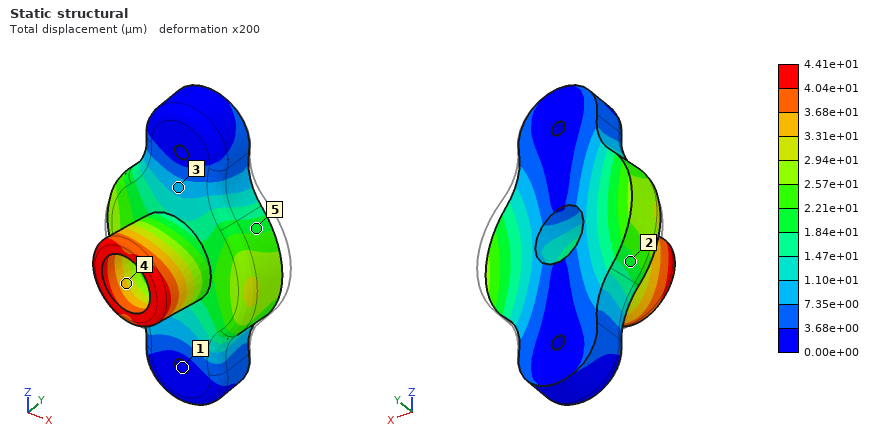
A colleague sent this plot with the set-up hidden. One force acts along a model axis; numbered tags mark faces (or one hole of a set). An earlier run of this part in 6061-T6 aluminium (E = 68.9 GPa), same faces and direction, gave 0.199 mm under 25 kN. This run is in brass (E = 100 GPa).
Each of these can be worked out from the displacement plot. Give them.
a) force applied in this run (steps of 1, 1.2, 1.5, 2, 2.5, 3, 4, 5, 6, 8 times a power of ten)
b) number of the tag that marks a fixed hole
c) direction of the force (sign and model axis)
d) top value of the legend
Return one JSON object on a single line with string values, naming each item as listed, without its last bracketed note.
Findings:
{"force applied in this run": "8 kN", "number of the tag that marks a fixed hole": "1", "direction of the force": "-X", "top value of the legend": "4.41e+01 µm"}
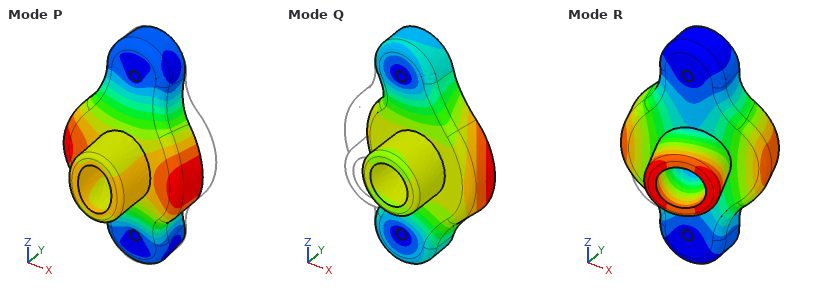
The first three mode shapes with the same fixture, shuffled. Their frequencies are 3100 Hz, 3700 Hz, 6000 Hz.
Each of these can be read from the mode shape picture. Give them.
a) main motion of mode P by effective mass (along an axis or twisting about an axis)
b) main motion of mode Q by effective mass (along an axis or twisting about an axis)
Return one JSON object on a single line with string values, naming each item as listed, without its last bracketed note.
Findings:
{"main motion of mode P by effective mass": "along Y", "main motion of mode Q by effective mass": "along X"}
